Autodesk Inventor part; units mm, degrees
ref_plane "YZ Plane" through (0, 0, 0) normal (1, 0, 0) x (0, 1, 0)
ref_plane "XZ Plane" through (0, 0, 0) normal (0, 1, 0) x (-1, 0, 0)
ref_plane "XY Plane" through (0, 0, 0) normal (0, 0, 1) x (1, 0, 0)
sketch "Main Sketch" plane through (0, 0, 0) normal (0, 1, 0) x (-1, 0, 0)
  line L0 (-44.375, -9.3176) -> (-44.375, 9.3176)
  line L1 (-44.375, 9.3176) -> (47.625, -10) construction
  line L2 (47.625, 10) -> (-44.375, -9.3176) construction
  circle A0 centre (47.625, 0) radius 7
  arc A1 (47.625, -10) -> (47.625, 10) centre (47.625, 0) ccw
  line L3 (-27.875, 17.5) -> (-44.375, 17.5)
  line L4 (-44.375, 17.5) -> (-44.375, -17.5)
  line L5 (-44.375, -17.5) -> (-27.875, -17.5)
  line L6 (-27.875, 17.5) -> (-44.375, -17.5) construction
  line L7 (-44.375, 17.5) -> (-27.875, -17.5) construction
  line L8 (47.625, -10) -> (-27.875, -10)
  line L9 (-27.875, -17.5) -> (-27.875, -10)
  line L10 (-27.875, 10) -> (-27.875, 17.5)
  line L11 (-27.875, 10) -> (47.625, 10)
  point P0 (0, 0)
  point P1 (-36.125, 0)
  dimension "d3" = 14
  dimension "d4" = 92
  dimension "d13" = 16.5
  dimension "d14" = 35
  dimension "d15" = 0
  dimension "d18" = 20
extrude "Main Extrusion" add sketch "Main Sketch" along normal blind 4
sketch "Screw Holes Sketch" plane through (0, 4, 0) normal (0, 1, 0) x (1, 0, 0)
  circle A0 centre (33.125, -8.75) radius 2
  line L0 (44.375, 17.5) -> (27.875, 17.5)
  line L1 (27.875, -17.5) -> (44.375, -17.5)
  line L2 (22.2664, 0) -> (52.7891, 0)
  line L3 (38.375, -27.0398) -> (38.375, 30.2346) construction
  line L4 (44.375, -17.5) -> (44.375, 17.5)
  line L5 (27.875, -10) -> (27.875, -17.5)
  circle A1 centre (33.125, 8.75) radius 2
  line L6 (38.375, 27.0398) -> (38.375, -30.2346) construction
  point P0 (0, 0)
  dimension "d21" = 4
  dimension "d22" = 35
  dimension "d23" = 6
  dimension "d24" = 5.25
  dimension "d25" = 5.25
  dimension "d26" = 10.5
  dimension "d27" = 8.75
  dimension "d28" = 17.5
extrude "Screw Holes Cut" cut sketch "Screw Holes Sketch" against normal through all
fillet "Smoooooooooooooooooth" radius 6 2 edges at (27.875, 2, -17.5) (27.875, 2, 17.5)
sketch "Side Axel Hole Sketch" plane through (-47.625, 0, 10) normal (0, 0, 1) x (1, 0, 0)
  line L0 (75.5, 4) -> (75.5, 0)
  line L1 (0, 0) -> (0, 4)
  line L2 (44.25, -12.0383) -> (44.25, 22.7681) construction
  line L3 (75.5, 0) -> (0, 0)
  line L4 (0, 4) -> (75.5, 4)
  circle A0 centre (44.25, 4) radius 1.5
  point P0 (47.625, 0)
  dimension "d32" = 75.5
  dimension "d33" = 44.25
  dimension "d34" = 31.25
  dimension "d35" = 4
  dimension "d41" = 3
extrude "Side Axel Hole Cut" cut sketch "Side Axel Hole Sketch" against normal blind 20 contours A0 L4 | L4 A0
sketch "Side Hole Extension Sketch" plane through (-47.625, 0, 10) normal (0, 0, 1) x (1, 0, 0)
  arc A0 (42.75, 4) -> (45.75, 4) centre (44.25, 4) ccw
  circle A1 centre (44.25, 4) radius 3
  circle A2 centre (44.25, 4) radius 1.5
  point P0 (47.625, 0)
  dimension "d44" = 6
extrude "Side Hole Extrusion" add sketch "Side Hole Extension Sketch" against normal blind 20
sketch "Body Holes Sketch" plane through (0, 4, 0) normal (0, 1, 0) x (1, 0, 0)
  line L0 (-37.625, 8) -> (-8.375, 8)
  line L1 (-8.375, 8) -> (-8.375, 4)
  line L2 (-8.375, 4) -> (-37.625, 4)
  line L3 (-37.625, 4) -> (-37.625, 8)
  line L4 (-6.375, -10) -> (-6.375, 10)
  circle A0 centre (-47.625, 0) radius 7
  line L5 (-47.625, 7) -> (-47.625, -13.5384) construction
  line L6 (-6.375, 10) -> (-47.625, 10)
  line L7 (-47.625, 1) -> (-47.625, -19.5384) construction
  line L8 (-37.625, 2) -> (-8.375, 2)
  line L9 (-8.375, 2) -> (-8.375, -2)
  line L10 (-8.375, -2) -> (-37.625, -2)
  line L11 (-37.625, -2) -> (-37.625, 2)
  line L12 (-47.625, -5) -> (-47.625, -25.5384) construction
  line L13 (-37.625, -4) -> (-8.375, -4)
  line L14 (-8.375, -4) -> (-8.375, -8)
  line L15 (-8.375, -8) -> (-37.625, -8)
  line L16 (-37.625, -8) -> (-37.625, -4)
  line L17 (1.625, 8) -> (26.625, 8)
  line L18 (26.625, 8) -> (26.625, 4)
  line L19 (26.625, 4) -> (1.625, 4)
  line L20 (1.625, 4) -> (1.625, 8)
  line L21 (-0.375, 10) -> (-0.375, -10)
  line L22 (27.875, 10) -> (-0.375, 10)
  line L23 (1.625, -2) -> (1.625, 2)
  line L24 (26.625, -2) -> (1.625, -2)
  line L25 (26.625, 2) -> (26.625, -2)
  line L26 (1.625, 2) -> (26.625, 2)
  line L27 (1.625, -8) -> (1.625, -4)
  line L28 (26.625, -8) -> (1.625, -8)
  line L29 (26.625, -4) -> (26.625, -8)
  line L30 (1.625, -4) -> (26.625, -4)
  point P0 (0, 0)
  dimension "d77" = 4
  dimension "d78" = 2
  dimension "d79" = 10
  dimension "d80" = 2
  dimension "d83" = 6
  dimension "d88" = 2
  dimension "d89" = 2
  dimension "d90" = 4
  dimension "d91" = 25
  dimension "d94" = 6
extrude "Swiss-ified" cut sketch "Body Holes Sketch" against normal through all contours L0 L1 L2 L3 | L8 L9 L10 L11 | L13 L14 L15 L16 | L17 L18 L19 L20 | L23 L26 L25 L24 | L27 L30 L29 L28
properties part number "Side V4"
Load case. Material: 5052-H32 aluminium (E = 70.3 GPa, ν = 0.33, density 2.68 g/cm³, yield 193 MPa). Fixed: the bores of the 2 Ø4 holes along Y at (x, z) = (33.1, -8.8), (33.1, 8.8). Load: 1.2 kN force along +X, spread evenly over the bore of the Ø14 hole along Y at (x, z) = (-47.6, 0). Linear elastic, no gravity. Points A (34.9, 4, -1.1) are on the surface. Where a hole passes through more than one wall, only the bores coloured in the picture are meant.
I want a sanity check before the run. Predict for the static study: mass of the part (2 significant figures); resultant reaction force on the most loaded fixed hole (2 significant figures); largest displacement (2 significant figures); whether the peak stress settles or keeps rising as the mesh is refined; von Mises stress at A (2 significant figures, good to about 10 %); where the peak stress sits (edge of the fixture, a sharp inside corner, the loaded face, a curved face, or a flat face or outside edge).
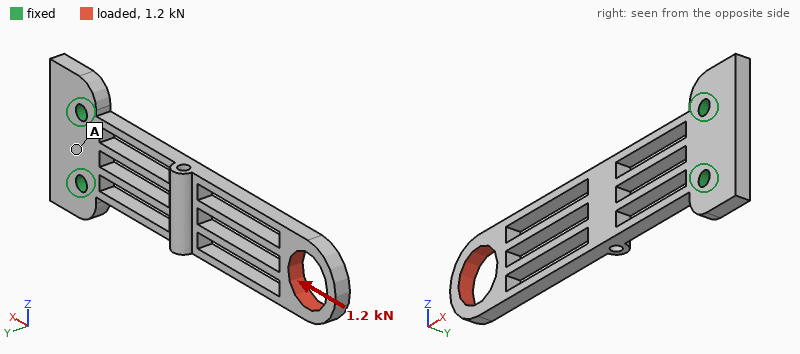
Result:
15 g
610 N
59 µm
keeps rising
5.9 MPa
a sharp inside corner
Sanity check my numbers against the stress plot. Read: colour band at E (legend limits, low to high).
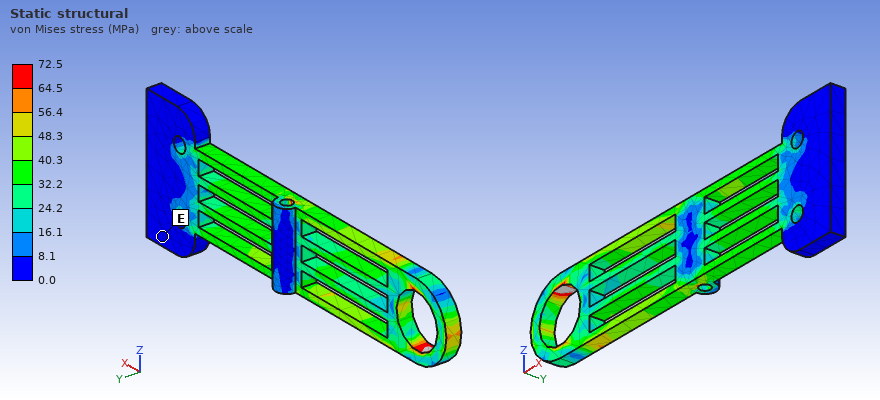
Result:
0.0 to 8.1 MPa
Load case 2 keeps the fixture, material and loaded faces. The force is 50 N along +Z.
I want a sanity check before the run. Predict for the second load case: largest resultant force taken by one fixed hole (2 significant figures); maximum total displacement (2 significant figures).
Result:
220 N
0.36 mm
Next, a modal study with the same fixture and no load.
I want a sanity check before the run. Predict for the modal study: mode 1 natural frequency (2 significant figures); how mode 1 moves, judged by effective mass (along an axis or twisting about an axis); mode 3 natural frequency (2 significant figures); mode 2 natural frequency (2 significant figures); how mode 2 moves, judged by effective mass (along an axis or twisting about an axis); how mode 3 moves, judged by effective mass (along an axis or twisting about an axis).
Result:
410 Hz
along Y
2100 Hz
970 Hz
along Z
twisting about X
